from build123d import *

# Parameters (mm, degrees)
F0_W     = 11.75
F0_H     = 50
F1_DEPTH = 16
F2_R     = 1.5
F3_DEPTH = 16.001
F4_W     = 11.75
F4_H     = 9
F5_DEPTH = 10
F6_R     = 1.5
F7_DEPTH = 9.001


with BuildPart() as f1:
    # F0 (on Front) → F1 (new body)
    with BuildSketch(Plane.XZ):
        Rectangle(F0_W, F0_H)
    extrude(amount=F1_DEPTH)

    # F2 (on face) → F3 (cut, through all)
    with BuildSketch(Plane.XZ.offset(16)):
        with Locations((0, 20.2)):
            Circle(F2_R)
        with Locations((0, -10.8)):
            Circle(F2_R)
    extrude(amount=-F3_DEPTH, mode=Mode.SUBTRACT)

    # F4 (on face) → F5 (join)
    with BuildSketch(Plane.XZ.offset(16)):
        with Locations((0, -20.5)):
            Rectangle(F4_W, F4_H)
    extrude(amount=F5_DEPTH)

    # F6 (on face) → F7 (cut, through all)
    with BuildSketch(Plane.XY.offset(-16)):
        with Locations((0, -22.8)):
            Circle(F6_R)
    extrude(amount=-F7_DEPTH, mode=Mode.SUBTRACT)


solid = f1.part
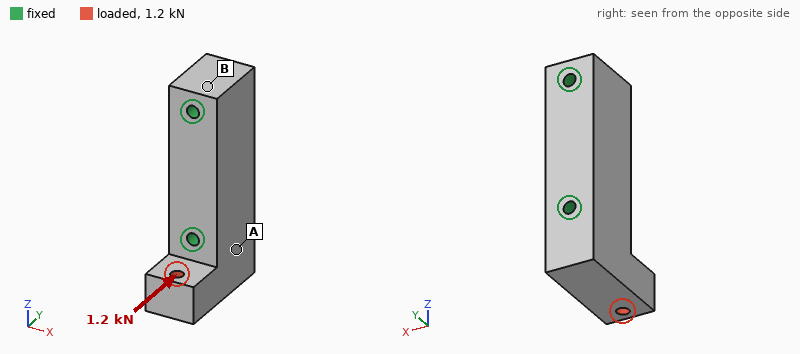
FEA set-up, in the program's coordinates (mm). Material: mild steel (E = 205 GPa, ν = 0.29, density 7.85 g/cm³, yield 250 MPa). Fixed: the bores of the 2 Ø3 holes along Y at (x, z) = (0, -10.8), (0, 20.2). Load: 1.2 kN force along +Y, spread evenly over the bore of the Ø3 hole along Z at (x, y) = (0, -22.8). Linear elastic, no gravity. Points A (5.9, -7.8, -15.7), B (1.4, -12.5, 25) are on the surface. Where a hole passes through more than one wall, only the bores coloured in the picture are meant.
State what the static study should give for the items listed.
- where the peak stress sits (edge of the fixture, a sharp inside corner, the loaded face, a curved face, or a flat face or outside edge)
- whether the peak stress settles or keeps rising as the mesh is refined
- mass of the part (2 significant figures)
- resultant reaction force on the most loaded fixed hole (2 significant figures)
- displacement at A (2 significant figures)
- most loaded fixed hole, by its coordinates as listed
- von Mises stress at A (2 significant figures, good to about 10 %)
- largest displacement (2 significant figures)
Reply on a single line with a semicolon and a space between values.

edge of the fixture; keeps rising; 80 g; 1.2 kN; 0.61 µm; (0, -10.8); 13 MPa; 3.9 µm
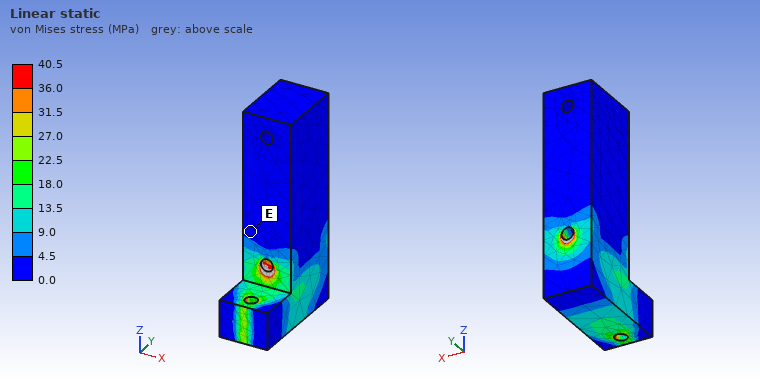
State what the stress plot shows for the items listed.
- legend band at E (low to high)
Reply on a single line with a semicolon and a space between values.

0.0 to 4.5 MPa
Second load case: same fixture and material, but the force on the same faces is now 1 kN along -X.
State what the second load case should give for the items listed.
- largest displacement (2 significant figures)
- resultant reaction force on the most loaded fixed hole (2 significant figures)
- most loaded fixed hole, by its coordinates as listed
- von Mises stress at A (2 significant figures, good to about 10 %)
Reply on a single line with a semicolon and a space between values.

13 µm; 1.2 kN; (0, -10.8); 38 MPa
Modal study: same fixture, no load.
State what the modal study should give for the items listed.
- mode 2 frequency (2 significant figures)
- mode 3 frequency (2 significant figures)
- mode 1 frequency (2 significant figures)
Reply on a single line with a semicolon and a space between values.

22 kHz; 27 kHz; 17 kHz
